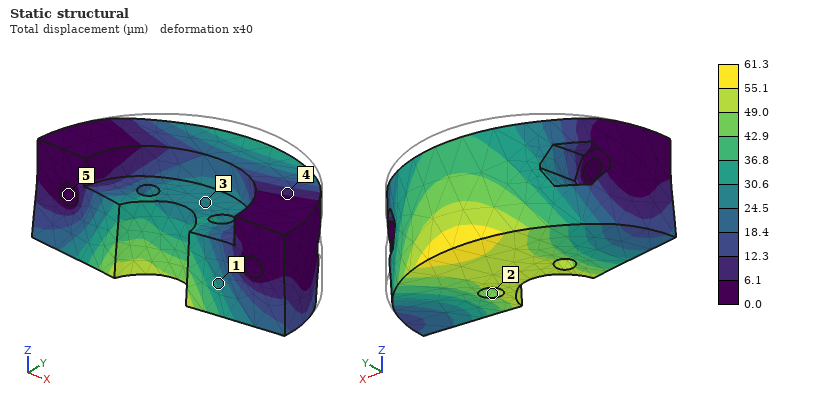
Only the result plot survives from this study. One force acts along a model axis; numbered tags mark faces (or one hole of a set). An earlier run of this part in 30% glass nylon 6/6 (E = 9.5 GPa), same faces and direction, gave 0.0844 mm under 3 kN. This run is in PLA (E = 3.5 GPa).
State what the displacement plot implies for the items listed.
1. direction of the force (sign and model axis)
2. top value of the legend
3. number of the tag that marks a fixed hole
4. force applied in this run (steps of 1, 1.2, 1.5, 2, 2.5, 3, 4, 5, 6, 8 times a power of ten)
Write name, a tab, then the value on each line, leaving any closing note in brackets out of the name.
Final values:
direction of the force	-Y
top value of the legend	61.3 µm
number of the tag that marks a fixed hole	5
force applied in this run	800 N
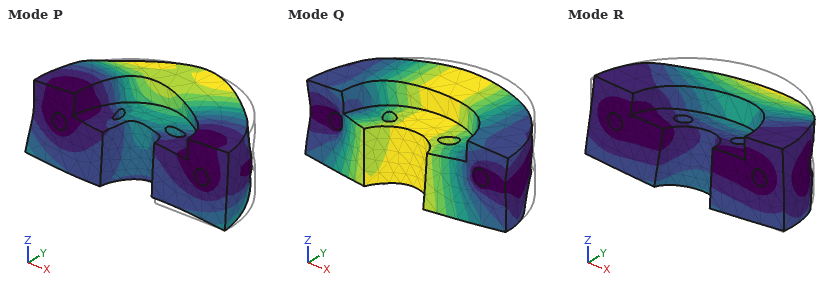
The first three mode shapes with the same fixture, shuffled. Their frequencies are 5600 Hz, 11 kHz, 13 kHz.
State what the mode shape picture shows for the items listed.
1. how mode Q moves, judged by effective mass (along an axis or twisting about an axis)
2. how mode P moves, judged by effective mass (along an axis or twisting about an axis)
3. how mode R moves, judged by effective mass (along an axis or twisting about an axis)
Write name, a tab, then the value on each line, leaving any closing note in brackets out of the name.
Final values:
how mode Q moves, judged by effective mass	along Y
how mode P moves, judged by effective mass	along X
how mode R moves, judged by effective mass	along Z
